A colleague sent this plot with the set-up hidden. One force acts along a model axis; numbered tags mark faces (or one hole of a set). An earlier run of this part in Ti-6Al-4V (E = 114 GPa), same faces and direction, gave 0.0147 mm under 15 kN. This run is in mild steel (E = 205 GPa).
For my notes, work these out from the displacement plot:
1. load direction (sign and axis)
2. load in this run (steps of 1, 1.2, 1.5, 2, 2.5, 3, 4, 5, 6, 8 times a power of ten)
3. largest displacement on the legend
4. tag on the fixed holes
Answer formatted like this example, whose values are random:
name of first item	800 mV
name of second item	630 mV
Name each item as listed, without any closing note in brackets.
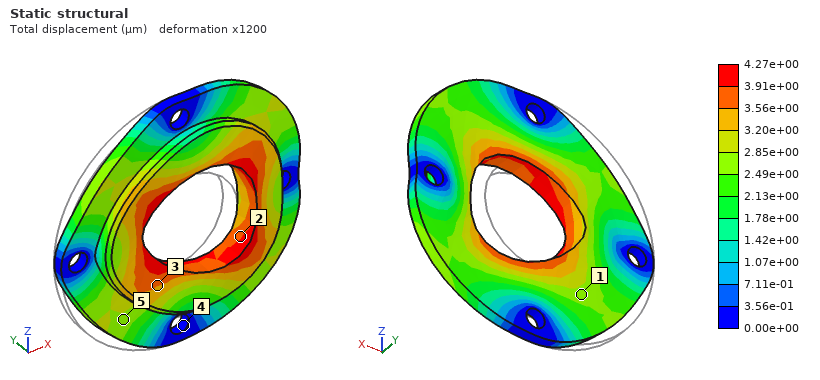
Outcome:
load direction	+X
load in this run	8 kN
largest displacement on the legend	4.27e+00 µm
tag on the fixed holes	4
